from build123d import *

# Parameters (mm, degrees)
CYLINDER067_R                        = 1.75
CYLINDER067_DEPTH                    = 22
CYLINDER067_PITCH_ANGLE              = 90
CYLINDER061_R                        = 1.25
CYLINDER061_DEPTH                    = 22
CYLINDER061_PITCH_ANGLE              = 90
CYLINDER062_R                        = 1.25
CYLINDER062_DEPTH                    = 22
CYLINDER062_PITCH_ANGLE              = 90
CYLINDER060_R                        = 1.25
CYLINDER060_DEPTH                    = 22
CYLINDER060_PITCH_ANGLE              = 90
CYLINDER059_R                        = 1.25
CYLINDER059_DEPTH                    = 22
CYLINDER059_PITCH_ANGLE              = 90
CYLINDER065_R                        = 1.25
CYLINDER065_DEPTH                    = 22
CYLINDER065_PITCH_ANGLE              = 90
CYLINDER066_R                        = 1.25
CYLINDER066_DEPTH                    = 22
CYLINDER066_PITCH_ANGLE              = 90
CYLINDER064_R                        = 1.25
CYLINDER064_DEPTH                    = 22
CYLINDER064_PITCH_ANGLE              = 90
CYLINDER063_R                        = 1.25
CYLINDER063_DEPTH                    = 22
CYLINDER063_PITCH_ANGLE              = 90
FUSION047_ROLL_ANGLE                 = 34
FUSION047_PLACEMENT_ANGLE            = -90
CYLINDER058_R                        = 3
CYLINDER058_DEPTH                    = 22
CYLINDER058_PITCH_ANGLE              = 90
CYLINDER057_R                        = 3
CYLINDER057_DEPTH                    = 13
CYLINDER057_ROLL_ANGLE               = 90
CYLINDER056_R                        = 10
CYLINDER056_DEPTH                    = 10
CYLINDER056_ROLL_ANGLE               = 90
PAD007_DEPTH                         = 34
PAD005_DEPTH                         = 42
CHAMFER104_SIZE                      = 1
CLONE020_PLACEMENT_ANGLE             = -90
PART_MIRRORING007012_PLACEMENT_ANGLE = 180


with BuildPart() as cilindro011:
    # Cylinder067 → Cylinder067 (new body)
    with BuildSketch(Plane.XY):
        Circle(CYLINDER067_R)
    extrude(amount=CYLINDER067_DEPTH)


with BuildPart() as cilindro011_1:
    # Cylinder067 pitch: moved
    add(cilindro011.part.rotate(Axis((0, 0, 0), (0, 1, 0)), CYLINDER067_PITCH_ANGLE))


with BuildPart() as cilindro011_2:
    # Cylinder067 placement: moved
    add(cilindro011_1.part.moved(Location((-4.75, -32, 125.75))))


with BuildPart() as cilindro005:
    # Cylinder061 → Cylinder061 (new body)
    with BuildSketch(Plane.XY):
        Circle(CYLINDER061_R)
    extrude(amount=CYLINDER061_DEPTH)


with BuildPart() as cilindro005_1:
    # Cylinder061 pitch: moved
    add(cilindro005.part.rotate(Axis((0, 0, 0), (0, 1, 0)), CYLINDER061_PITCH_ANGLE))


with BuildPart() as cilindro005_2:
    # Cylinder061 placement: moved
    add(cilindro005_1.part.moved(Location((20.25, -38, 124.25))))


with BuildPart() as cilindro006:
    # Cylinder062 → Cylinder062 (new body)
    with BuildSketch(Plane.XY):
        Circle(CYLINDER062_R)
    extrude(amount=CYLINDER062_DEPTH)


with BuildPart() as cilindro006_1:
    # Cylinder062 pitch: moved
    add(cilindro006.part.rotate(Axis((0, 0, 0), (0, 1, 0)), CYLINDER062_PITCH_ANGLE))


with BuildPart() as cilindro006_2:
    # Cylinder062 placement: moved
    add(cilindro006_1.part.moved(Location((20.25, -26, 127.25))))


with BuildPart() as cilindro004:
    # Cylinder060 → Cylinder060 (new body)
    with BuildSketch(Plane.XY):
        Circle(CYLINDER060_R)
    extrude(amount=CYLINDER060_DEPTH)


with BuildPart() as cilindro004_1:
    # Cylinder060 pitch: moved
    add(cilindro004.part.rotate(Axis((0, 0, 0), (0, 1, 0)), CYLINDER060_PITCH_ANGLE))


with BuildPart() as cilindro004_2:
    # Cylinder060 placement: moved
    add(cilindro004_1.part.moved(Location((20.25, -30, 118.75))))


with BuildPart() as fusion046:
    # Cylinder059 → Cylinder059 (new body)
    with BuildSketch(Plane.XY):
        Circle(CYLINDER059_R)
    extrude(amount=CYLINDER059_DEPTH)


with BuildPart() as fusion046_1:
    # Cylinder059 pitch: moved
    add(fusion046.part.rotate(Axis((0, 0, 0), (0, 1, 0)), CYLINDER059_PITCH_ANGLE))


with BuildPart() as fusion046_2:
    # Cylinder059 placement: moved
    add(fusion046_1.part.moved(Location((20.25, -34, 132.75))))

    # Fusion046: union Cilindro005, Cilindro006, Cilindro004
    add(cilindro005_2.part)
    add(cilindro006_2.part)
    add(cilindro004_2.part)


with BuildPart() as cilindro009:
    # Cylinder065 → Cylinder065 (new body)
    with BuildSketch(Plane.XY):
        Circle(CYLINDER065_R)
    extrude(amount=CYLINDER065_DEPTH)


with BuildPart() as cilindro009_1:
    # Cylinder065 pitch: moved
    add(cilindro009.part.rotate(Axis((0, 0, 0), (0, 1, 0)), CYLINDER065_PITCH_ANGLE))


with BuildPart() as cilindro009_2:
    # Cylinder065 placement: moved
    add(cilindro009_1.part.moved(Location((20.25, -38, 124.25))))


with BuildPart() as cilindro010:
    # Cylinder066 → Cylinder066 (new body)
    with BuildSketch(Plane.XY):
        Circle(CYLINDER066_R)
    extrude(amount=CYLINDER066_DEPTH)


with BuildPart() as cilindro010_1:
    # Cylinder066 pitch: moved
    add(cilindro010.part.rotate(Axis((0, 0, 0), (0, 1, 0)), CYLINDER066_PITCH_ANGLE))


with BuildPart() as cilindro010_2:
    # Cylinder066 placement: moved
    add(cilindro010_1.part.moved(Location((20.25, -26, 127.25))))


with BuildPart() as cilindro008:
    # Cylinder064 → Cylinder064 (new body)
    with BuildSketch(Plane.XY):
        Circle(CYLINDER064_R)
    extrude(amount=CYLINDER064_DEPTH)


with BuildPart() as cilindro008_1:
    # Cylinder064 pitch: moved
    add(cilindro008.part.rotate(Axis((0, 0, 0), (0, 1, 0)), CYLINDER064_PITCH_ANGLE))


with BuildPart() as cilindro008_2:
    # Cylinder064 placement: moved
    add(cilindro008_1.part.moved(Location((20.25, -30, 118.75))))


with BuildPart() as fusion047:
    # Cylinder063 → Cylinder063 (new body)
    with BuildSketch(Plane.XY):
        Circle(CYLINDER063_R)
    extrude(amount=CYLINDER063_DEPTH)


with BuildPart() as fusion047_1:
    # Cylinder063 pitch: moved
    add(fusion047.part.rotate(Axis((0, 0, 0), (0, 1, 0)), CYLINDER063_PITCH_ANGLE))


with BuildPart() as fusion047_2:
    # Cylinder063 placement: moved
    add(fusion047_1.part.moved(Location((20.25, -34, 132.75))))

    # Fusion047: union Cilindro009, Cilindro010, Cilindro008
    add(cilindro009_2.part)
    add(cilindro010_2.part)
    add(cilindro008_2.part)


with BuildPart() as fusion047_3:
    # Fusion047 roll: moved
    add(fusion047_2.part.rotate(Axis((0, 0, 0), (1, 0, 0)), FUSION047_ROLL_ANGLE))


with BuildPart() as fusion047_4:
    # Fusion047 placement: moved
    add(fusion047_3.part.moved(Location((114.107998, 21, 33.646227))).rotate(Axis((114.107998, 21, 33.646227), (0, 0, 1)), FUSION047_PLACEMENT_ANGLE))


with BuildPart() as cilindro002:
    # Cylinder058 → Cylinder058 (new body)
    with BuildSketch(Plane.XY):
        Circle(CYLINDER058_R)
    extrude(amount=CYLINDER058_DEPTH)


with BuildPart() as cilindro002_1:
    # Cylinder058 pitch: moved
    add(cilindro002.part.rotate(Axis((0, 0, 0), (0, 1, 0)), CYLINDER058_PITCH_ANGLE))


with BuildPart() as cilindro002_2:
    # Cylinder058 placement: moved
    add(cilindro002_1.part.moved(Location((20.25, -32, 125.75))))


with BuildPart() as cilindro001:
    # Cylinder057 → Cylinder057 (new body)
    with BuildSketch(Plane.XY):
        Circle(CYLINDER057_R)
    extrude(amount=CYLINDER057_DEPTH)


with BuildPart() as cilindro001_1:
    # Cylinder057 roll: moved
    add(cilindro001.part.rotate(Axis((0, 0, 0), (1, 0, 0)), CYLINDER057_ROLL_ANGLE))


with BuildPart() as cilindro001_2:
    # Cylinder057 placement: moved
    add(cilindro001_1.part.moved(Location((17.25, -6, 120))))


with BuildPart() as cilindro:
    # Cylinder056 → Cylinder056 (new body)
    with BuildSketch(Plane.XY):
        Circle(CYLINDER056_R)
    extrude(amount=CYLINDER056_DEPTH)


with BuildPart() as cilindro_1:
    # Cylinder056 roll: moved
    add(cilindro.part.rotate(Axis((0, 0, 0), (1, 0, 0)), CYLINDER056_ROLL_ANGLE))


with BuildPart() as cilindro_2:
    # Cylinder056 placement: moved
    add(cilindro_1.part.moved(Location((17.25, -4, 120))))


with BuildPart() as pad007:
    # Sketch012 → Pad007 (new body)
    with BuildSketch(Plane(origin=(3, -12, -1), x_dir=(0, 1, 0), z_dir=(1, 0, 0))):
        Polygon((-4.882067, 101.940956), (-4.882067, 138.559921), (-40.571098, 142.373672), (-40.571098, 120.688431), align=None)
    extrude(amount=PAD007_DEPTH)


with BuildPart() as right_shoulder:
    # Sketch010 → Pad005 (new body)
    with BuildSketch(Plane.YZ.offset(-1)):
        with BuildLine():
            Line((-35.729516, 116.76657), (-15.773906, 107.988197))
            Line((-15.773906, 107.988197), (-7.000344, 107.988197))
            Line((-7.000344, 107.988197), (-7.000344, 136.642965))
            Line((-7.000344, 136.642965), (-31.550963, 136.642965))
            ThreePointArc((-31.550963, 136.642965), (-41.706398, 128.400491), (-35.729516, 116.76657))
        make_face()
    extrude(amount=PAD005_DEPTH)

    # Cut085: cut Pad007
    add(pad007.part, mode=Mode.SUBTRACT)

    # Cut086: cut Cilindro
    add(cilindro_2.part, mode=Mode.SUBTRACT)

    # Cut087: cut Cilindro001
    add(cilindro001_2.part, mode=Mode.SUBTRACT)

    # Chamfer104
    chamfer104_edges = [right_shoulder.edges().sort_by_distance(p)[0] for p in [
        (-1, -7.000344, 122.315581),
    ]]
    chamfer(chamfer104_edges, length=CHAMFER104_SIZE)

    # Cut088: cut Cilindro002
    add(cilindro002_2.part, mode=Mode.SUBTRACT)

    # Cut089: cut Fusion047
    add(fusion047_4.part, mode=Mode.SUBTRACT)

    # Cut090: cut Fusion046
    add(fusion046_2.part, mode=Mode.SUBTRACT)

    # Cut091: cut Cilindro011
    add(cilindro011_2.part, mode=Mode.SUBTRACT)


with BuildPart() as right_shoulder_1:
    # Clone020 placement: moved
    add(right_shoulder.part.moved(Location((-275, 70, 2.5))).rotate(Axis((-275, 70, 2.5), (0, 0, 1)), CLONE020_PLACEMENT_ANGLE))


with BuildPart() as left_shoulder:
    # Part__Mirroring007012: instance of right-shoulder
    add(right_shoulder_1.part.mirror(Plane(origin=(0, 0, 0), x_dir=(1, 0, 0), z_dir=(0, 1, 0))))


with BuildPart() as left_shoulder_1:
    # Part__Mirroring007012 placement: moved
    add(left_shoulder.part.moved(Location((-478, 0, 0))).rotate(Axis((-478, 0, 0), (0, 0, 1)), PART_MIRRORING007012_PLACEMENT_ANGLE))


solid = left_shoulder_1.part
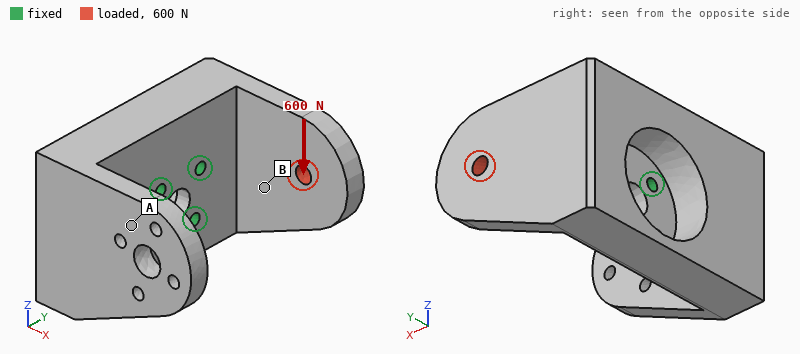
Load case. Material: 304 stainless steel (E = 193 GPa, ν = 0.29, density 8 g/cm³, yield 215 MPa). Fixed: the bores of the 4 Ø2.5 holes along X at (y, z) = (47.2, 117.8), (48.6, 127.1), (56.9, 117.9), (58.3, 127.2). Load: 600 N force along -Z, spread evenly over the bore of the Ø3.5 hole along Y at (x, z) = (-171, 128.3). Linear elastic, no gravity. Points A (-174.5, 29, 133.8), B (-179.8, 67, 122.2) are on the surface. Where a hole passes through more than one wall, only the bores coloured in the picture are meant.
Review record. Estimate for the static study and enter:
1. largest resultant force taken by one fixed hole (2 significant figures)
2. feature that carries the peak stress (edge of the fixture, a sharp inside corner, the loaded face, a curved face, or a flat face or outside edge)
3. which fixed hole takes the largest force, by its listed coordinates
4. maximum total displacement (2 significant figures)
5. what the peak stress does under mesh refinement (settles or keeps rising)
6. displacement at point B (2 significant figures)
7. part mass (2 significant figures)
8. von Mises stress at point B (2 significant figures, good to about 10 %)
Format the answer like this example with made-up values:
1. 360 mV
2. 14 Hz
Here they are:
1. 750 N
2. edge of the fixture
3. (58.3, 127.2)
4. 23 µm
5. keeps rising
6. 8.2 µm
7. 110 g
8. 17 MPa
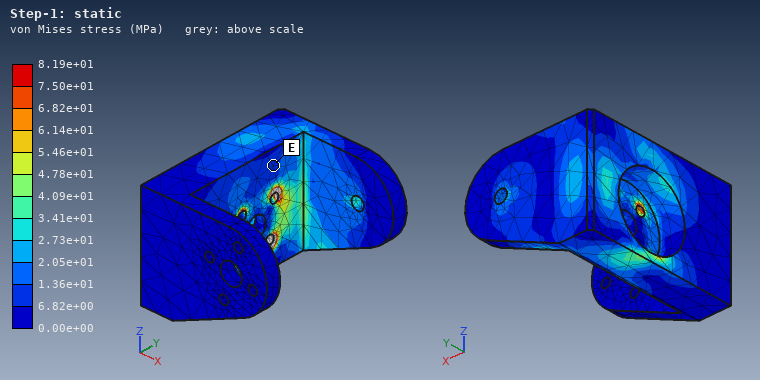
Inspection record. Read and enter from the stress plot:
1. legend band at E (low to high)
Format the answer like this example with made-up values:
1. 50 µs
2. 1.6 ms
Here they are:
1. 6.82e+00 to 1.36e+01 MPa
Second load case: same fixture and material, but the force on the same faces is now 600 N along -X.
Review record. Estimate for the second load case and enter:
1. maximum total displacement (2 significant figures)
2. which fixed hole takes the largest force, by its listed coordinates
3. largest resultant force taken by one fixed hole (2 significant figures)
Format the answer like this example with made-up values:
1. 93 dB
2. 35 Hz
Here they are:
1. 17 µm
2. (58.3, 127.2)
3. 750 N
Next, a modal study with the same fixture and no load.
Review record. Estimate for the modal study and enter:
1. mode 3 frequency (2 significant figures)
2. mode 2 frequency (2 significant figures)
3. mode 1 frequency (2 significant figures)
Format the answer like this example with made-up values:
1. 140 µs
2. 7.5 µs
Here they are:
1. 6200 Hz
2. 4800 Hz
3. 3900 Hz
